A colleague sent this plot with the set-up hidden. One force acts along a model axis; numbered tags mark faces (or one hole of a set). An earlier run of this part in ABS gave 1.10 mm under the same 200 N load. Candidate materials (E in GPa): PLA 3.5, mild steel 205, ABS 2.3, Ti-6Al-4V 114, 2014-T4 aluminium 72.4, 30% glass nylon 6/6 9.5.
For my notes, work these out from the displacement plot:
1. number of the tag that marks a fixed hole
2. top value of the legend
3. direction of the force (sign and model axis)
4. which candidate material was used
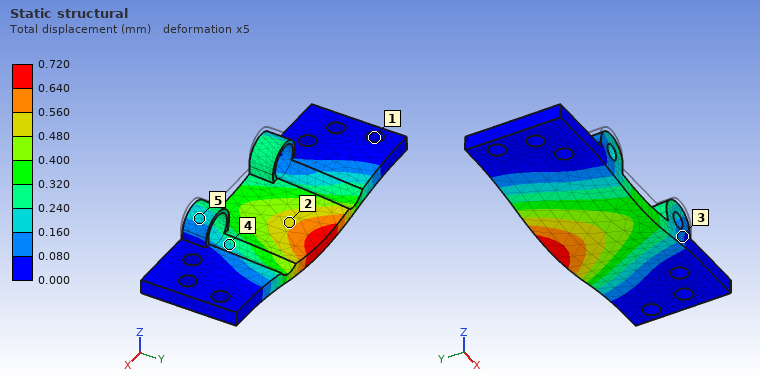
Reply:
1
0.720 mm
-Z
PLA
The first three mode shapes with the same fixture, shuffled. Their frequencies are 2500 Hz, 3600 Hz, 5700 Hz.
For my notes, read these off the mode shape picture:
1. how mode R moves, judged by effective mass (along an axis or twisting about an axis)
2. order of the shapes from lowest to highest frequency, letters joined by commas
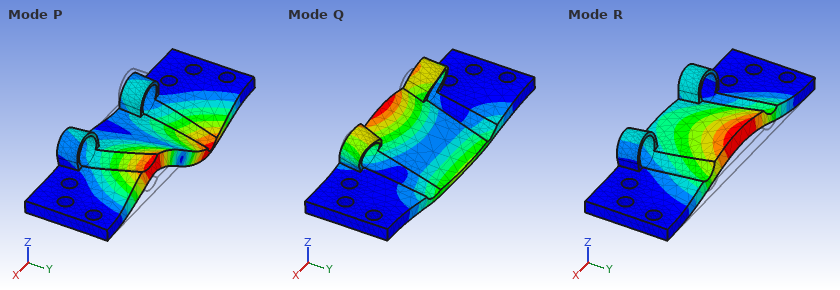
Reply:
along Z
R, Q, P
